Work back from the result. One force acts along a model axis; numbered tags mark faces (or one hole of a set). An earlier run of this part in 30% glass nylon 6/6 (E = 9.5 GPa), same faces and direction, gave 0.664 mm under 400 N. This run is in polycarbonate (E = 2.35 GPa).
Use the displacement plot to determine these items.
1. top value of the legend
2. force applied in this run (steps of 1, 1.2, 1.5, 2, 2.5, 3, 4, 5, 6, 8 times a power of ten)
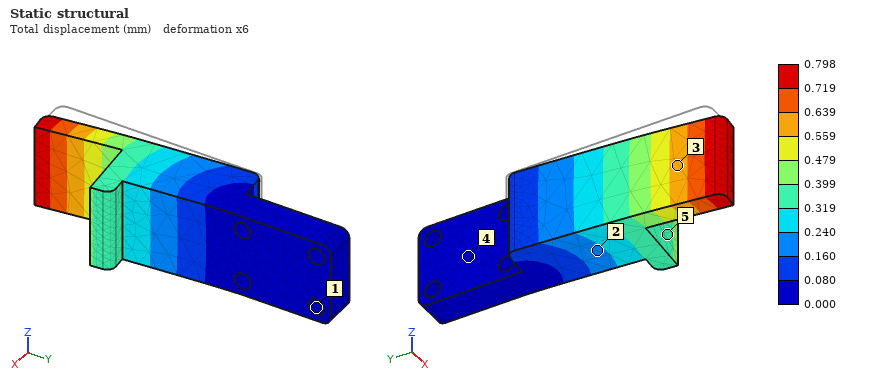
0.798 mm
120 N
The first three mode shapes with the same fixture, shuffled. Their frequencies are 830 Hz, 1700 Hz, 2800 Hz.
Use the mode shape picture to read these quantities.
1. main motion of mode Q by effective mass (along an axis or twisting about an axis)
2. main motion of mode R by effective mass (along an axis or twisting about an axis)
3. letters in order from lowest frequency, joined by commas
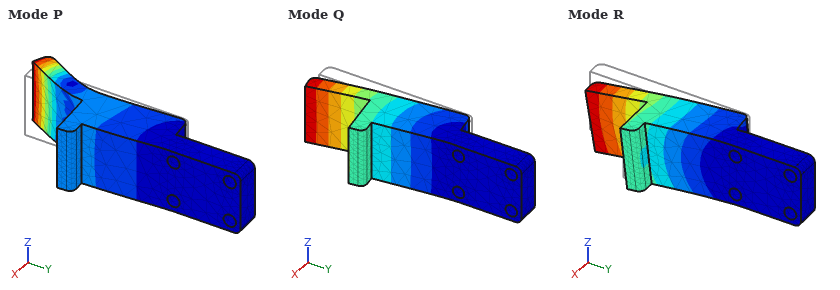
along X
along Z
Q, R, P
